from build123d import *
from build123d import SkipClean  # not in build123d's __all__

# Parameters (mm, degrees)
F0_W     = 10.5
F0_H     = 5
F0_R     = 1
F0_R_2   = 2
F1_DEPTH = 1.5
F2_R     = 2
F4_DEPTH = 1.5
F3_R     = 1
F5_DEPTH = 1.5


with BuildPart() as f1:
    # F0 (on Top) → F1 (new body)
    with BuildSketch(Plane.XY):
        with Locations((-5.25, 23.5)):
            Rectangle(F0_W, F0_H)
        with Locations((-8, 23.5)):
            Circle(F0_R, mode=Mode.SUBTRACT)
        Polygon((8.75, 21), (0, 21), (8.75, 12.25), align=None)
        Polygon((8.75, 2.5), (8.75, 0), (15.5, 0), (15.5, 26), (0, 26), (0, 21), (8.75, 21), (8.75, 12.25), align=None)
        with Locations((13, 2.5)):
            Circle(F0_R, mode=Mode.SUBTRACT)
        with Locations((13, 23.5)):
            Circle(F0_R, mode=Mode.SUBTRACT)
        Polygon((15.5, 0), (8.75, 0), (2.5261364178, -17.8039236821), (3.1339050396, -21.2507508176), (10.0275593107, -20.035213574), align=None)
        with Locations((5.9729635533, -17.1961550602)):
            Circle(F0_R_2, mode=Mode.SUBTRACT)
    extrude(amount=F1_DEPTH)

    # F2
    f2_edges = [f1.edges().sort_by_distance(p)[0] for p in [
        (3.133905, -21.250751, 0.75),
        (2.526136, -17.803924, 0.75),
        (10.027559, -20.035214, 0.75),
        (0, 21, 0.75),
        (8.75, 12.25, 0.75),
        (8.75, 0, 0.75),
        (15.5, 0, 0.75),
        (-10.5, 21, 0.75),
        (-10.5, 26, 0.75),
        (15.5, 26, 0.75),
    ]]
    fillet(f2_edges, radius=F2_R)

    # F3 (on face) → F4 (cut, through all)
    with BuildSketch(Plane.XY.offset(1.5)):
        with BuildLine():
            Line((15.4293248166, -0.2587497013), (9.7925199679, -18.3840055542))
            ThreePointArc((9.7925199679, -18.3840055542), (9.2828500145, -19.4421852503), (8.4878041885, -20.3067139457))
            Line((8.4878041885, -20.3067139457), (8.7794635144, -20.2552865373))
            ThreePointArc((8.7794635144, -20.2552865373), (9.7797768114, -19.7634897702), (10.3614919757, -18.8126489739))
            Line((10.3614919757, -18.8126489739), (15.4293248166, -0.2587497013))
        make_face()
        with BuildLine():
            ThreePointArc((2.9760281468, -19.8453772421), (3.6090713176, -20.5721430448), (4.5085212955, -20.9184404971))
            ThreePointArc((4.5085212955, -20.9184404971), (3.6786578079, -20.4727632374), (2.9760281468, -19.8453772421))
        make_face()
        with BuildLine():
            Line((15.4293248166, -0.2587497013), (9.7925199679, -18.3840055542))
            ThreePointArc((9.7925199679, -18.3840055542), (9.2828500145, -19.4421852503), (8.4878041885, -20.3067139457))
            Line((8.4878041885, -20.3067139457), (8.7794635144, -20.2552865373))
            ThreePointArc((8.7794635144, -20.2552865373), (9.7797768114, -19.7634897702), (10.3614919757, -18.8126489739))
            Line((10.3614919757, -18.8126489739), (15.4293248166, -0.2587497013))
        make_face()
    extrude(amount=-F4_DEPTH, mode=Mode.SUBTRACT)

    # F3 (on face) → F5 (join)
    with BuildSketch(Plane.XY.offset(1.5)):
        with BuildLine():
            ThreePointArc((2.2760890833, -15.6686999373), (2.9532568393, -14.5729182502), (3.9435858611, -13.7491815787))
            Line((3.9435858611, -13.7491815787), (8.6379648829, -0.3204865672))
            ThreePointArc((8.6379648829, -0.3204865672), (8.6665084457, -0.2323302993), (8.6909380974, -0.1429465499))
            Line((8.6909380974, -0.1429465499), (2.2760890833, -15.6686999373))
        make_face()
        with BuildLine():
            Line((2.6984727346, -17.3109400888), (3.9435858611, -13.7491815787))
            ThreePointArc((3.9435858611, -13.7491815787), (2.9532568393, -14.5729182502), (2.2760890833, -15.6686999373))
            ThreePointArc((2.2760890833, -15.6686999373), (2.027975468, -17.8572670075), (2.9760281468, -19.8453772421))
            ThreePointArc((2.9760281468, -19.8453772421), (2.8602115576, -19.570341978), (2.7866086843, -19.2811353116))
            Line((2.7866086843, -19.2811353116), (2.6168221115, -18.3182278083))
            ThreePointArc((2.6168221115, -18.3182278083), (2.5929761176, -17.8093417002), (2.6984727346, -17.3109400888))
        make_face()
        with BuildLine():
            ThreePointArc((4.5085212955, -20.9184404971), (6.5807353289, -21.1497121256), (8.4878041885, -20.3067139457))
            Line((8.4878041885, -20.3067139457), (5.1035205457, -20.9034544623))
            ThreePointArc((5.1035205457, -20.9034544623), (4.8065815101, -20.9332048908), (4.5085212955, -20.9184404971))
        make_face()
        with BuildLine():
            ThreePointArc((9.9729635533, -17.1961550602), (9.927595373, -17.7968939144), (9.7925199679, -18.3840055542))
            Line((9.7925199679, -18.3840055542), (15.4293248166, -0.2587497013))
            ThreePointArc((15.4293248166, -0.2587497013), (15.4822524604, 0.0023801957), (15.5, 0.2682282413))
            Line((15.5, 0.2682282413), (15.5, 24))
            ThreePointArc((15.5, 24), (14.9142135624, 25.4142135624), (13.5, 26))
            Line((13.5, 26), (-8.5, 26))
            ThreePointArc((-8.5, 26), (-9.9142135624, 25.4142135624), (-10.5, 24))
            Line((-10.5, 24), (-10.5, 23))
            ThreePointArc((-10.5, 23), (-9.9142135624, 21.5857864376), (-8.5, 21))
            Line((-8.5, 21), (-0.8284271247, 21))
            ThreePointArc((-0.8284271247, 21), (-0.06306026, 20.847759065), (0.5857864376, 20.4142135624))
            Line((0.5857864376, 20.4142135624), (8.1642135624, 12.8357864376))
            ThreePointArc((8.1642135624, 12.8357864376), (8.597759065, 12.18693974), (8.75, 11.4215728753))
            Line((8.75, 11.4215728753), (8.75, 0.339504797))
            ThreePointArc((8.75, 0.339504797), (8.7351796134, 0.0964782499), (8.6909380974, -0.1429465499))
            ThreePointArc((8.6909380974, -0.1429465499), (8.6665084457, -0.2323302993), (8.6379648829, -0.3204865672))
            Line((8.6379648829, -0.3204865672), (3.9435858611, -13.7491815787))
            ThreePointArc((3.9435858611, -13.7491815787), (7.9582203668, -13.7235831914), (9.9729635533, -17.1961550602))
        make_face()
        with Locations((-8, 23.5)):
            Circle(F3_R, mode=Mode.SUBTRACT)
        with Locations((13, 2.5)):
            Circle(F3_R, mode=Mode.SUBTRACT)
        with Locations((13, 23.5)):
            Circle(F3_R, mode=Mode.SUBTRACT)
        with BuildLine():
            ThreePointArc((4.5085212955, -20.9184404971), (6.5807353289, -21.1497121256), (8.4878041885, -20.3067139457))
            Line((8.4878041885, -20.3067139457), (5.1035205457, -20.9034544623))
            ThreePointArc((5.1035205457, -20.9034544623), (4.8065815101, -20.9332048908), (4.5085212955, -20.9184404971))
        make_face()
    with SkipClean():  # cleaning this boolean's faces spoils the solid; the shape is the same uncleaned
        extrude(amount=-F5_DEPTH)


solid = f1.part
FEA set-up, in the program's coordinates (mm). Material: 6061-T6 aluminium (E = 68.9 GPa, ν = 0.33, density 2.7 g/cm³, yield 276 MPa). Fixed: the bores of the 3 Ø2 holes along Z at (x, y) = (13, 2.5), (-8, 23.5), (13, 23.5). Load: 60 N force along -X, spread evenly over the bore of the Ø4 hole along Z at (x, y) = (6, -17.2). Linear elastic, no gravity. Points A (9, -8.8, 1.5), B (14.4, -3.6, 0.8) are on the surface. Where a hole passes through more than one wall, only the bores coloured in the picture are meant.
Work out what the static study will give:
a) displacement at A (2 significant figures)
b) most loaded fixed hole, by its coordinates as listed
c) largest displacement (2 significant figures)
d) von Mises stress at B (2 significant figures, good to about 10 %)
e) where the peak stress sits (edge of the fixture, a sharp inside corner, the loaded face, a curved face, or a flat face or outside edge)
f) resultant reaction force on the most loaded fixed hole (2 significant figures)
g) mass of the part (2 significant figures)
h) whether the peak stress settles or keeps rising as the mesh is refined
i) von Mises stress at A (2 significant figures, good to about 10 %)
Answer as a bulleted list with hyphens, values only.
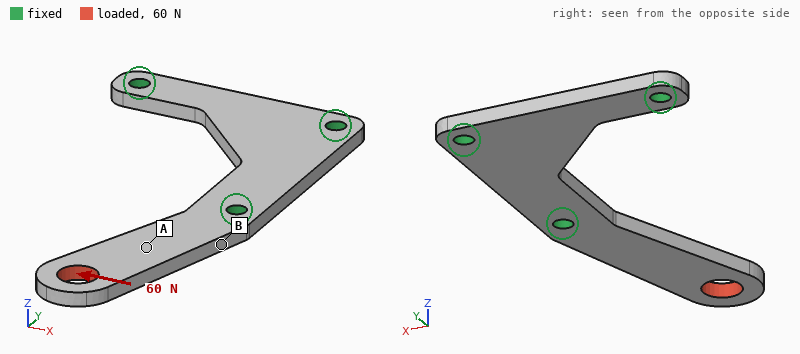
- 0.041 mm
- (13, 2.5)
- 0.11 mm
- 81 MPa
- edge of the fixture
- 100 N
- 1.8 g
- keeps rising
- 15 MPa
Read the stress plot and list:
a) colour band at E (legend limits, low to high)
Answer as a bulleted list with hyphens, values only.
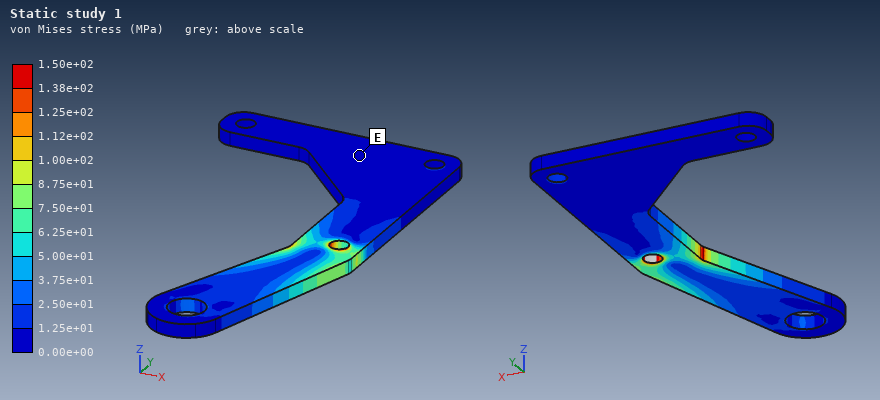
- 0.00e+00 to 1.25e+01 MPa
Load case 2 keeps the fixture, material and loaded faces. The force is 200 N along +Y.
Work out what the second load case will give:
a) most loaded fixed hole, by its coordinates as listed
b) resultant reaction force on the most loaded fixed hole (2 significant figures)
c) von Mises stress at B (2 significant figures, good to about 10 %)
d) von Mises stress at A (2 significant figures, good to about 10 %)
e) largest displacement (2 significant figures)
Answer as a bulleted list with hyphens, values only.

- (13, 2.5)
- 150 N
- 76 MPa
- 25 MPa
- 0.13 mm
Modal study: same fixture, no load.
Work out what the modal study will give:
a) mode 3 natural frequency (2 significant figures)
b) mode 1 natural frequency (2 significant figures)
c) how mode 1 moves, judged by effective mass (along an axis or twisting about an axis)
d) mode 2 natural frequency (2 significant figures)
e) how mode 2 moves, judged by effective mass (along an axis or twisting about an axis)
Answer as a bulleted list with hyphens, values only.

- 12 kHz
- 2300 Hz
- along Z
- 7900 Hz
- along X
